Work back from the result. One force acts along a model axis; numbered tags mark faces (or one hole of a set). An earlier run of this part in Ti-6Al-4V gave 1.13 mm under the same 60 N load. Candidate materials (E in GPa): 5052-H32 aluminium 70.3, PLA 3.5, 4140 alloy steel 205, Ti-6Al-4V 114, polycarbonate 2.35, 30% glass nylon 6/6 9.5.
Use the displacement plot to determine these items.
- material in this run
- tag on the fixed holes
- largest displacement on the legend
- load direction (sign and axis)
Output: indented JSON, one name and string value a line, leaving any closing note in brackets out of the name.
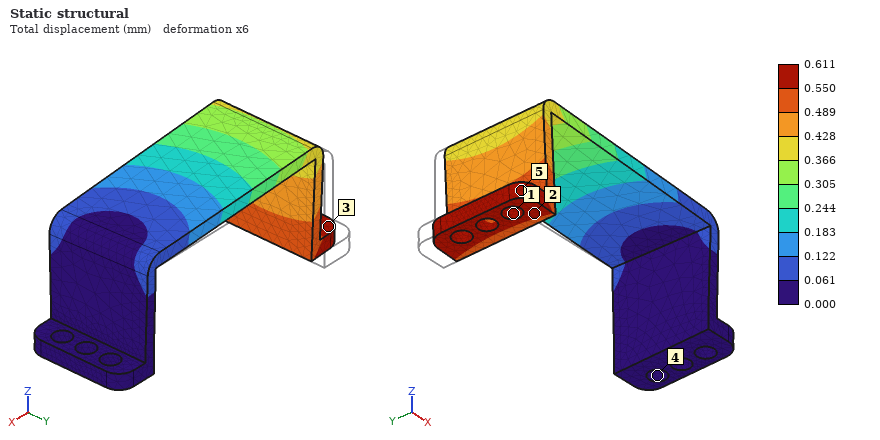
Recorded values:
{
  "material in this run": "4140 alloy steel",
  "tag on the fixed holes": "4",
  "largest displacement on the legend": "0.611 mm",
  "load direction": "-Y"
}
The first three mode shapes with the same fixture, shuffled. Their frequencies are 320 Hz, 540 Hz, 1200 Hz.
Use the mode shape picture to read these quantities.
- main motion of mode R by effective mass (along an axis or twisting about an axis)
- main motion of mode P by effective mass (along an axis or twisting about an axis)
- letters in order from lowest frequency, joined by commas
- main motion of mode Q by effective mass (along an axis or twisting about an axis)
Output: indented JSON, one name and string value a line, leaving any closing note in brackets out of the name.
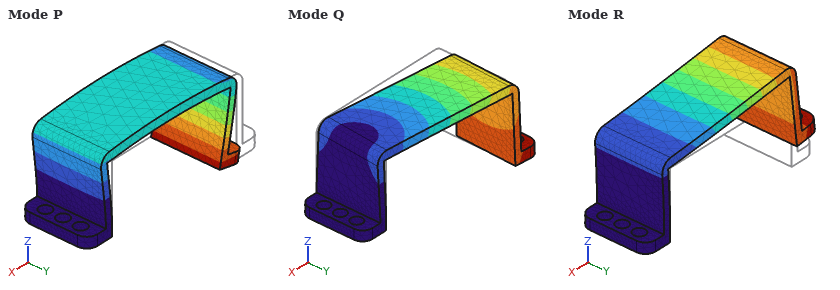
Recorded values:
{
  "main motion of mode R by effective mass": "along Z",
  "main motion of mode P by effective mass": "along X",
  "letters in order from lowest frequency, joined by commas": "R, Q, P",
  "main motion of mode Q by effective mass": "along Y"
}
